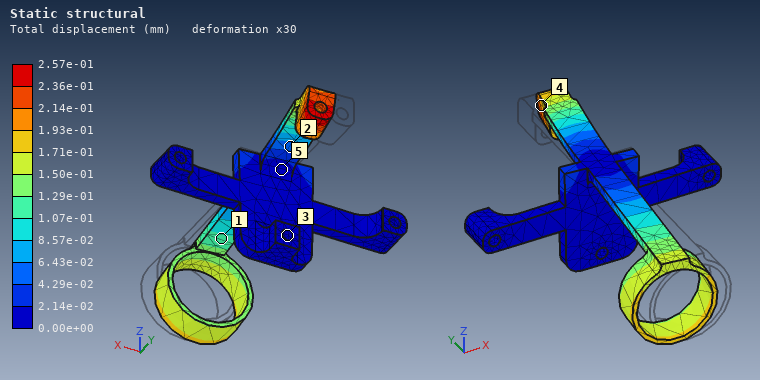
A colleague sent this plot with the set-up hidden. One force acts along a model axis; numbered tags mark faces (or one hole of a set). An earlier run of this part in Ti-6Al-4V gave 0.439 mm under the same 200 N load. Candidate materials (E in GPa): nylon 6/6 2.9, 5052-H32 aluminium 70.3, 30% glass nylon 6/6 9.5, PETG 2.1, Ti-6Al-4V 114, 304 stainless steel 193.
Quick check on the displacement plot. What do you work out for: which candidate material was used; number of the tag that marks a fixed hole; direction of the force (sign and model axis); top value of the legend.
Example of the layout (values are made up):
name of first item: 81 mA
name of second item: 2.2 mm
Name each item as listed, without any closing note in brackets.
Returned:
which candidate material was used: 304 stainless steel
number of the tag that marks a fixed hole: 3
direction of the force: +X
top value of the legend: 2.57e-01 mm
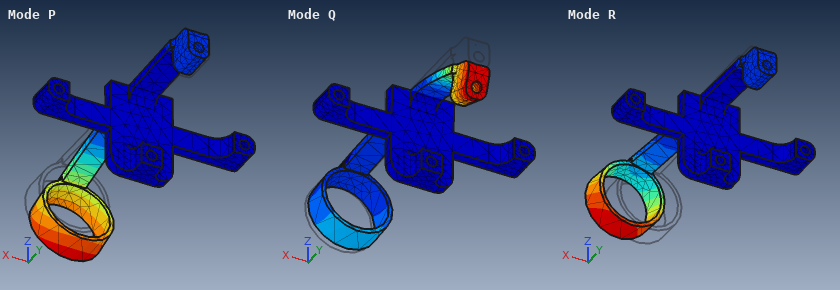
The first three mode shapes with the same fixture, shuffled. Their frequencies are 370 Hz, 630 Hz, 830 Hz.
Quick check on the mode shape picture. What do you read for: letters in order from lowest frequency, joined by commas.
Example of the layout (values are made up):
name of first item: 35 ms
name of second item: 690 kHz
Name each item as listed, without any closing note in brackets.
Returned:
letters in order from lowest frequency, joined by commas: P, R, Q
